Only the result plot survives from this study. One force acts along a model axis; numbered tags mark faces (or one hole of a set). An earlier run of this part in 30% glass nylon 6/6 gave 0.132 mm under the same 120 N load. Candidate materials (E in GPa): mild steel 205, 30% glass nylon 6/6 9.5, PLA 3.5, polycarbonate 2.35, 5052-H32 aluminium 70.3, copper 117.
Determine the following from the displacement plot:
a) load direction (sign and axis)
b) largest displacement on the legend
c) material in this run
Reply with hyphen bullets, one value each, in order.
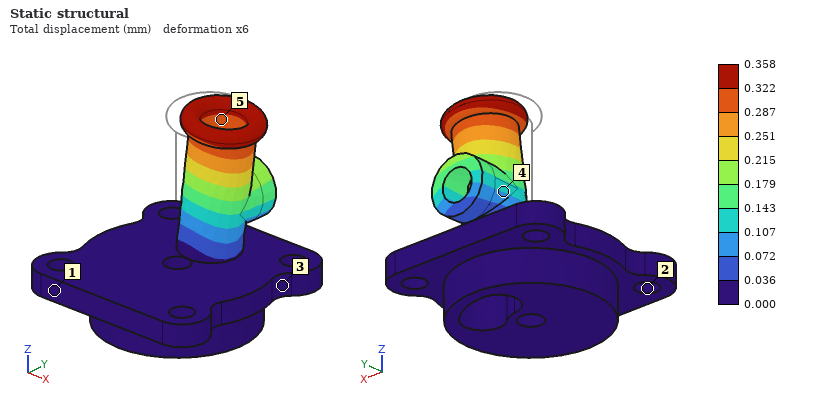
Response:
- +X
- 0.358 mm
- PLA
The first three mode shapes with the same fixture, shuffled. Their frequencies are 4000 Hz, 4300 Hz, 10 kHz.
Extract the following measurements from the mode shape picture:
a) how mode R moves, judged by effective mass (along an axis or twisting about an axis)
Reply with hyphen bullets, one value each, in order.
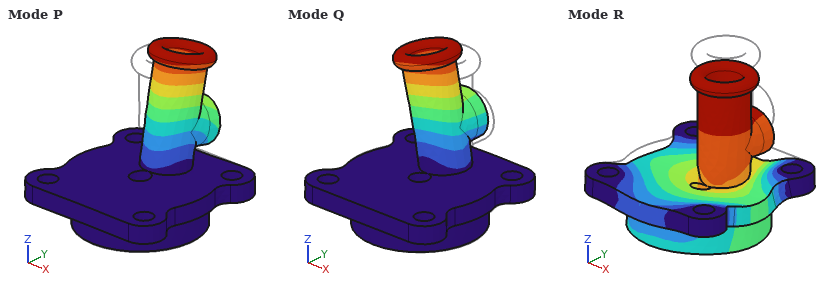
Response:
- along Z
